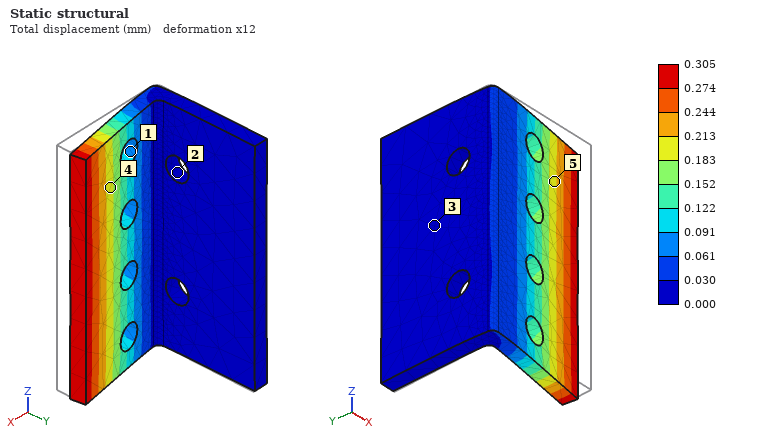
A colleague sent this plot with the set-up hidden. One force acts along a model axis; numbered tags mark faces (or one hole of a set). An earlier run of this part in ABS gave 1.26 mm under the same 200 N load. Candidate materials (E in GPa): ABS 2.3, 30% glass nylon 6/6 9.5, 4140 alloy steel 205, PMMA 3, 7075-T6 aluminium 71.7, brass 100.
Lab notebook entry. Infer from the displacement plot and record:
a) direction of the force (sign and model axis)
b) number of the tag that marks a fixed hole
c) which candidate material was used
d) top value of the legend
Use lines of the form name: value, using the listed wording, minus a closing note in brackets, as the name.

direction of the force: +Y
number of the tag that marks a fixed hole: 2
which candidate material was used: 30% glass nylon 6/6
top value of the legend: 0.305 mm
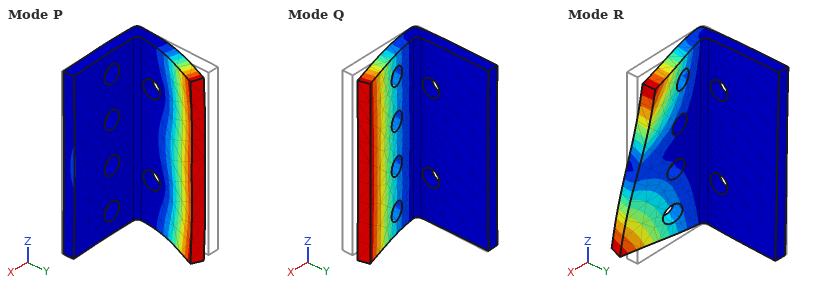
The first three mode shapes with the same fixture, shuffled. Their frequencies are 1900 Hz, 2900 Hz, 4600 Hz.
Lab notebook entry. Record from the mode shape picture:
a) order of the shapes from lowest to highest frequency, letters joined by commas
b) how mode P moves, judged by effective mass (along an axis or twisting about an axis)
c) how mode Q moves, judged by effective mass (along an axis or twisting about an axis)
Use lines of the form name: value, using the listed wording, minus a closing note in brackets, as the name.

order of the shapes from lowest to highest frequency, letters joined by commas: Q, R, P
how mode P moves, judged by effective mass: along X
how mode Q moves, judged by effective mass: along Y
